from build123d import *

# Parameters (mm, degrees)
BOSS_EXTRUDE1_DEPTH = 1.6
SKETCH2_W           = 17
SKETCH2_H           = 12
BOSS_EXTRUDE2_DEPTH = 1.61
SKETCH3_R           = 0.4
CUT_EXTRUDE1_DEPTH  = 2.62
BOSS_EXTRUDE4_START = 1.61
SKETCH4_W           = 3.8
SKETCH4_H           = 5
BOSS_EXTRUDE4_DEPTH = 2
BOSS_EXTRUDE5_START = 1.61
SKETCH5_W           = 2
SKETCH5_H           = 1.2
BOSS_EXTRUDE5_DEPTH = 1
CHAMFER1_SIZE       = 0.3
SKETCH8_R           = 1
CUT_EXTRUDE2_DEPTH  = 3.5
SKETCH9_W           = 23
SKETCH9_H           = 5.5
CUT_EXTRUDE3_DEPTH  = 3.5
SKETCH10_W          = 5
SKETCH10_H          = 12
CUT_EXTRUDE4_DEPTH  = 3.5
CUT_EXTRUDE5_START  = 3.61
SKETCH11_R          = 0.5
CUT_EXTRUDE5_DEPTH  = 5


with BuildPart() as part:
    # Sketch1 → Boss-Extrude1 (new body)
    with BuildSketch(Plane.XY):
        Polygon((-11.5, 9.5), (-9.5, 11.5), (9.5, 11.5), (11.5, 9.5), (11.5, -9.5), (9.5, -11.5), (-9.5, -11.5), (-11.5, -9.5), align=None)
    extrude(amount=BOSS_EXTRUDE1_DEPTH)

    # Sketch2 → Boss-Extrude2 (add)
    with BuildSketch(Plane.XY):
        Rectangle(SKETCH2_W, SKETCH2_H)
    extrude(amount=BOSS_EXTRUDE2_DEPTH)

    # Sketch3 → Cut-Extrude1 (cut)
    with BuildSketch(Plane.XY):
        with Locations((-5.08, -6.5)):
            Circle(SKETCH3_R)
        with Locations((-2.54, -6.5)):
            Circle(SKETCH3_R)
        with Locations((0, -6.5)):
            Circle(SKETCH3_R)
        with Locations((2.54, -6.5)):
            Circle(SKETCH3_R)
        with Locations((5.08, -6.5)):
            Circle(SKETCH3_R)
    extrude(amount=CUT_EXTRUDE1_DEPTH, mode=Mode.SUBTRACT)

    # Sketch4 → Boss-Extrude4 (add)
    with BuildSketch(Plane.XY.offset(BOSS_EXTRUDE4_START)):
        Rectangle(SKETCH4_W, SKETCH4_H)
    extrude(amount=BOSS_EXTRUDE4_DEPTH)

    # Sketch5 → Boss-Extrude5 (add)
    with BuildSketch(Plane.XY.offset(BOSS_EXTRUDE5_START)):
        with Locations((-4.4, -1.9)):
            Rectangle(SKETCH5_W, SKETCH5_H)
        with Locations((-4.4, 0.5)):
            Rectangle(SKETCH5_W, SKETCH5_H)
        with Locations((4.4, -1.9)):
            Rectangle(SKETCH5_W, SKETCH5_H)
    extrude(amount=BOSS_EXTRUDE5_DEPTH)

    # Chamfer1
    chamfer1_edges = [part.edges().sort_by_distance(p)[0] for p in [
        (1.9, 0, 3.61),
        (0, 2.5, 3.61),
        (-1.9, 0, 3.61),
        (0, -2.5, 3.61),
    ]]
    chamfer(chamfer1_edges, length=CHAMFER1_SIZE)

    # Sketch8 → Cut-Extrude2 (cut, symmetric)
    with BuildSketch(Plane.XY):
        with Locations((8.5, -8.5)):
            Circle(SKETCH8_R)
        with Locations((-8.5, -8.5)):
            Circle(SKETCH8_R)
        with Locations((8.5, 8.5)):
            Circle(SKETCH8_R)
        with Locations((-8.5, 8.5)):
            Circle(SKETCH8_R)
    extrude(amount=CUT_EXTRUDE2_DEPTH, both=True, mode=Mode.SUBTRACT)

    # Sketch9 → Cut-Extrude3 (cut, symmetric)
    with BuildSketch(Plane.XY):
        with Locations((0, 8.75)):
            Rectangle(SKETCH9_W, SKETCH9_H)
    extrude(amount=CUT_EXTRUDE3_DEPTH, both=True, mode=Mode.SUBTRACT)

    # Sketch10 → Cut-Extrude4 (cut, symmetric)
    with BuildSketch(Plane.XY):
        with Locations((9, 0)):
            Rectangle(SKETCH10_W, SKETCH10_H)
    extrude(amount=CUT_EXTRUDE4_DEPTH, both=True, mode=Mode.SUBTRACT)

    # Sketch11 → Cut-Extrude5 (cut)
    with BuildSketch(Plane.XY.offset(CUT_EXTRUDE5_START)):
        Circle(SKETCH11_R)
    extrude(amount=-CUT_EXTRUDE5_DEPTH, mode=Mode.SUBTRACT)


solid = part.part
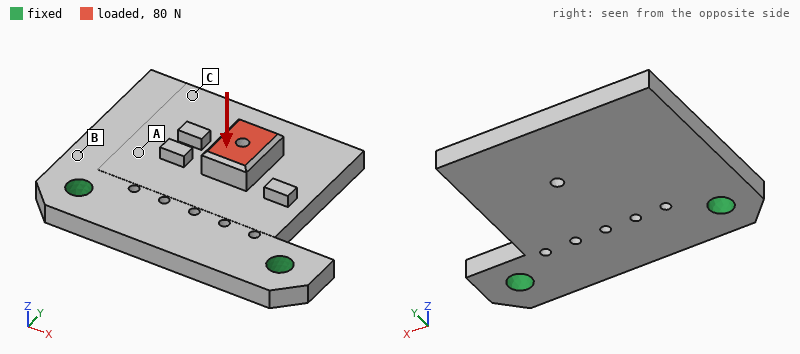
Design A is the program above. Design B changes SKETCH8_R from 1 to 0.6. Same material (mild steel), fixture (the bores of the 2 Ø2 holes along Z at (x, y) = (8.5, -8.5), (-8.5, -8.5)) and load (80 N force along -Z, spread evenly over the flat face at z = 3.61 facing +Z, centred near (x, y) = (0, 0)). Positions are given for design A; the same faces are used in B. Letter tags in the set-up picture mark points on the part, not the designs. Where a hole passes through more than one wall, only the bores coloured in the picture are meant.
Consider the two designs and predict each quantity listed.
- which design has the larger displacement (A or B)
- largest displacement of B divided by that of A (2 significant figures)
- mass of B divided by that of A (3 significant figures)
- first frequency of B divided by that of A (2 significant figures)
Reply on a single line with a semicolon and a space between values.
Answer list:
B; 1.2; 1.01; 0.91
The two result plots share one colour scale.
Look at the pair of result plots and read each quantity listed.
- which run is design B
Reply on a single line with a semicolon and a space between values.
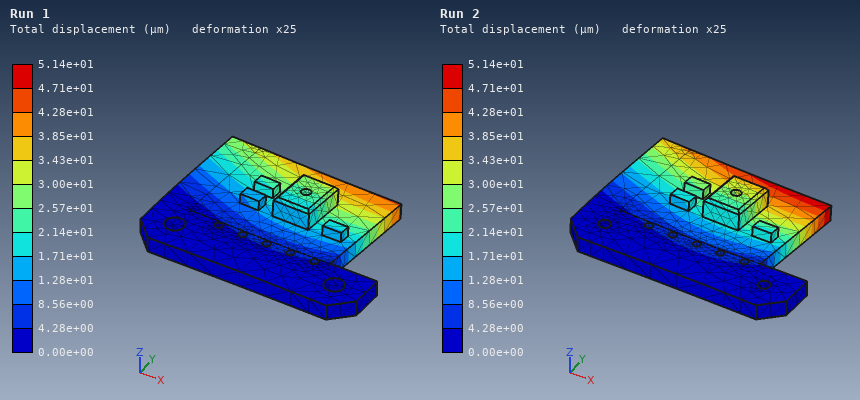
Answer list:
Run 2
